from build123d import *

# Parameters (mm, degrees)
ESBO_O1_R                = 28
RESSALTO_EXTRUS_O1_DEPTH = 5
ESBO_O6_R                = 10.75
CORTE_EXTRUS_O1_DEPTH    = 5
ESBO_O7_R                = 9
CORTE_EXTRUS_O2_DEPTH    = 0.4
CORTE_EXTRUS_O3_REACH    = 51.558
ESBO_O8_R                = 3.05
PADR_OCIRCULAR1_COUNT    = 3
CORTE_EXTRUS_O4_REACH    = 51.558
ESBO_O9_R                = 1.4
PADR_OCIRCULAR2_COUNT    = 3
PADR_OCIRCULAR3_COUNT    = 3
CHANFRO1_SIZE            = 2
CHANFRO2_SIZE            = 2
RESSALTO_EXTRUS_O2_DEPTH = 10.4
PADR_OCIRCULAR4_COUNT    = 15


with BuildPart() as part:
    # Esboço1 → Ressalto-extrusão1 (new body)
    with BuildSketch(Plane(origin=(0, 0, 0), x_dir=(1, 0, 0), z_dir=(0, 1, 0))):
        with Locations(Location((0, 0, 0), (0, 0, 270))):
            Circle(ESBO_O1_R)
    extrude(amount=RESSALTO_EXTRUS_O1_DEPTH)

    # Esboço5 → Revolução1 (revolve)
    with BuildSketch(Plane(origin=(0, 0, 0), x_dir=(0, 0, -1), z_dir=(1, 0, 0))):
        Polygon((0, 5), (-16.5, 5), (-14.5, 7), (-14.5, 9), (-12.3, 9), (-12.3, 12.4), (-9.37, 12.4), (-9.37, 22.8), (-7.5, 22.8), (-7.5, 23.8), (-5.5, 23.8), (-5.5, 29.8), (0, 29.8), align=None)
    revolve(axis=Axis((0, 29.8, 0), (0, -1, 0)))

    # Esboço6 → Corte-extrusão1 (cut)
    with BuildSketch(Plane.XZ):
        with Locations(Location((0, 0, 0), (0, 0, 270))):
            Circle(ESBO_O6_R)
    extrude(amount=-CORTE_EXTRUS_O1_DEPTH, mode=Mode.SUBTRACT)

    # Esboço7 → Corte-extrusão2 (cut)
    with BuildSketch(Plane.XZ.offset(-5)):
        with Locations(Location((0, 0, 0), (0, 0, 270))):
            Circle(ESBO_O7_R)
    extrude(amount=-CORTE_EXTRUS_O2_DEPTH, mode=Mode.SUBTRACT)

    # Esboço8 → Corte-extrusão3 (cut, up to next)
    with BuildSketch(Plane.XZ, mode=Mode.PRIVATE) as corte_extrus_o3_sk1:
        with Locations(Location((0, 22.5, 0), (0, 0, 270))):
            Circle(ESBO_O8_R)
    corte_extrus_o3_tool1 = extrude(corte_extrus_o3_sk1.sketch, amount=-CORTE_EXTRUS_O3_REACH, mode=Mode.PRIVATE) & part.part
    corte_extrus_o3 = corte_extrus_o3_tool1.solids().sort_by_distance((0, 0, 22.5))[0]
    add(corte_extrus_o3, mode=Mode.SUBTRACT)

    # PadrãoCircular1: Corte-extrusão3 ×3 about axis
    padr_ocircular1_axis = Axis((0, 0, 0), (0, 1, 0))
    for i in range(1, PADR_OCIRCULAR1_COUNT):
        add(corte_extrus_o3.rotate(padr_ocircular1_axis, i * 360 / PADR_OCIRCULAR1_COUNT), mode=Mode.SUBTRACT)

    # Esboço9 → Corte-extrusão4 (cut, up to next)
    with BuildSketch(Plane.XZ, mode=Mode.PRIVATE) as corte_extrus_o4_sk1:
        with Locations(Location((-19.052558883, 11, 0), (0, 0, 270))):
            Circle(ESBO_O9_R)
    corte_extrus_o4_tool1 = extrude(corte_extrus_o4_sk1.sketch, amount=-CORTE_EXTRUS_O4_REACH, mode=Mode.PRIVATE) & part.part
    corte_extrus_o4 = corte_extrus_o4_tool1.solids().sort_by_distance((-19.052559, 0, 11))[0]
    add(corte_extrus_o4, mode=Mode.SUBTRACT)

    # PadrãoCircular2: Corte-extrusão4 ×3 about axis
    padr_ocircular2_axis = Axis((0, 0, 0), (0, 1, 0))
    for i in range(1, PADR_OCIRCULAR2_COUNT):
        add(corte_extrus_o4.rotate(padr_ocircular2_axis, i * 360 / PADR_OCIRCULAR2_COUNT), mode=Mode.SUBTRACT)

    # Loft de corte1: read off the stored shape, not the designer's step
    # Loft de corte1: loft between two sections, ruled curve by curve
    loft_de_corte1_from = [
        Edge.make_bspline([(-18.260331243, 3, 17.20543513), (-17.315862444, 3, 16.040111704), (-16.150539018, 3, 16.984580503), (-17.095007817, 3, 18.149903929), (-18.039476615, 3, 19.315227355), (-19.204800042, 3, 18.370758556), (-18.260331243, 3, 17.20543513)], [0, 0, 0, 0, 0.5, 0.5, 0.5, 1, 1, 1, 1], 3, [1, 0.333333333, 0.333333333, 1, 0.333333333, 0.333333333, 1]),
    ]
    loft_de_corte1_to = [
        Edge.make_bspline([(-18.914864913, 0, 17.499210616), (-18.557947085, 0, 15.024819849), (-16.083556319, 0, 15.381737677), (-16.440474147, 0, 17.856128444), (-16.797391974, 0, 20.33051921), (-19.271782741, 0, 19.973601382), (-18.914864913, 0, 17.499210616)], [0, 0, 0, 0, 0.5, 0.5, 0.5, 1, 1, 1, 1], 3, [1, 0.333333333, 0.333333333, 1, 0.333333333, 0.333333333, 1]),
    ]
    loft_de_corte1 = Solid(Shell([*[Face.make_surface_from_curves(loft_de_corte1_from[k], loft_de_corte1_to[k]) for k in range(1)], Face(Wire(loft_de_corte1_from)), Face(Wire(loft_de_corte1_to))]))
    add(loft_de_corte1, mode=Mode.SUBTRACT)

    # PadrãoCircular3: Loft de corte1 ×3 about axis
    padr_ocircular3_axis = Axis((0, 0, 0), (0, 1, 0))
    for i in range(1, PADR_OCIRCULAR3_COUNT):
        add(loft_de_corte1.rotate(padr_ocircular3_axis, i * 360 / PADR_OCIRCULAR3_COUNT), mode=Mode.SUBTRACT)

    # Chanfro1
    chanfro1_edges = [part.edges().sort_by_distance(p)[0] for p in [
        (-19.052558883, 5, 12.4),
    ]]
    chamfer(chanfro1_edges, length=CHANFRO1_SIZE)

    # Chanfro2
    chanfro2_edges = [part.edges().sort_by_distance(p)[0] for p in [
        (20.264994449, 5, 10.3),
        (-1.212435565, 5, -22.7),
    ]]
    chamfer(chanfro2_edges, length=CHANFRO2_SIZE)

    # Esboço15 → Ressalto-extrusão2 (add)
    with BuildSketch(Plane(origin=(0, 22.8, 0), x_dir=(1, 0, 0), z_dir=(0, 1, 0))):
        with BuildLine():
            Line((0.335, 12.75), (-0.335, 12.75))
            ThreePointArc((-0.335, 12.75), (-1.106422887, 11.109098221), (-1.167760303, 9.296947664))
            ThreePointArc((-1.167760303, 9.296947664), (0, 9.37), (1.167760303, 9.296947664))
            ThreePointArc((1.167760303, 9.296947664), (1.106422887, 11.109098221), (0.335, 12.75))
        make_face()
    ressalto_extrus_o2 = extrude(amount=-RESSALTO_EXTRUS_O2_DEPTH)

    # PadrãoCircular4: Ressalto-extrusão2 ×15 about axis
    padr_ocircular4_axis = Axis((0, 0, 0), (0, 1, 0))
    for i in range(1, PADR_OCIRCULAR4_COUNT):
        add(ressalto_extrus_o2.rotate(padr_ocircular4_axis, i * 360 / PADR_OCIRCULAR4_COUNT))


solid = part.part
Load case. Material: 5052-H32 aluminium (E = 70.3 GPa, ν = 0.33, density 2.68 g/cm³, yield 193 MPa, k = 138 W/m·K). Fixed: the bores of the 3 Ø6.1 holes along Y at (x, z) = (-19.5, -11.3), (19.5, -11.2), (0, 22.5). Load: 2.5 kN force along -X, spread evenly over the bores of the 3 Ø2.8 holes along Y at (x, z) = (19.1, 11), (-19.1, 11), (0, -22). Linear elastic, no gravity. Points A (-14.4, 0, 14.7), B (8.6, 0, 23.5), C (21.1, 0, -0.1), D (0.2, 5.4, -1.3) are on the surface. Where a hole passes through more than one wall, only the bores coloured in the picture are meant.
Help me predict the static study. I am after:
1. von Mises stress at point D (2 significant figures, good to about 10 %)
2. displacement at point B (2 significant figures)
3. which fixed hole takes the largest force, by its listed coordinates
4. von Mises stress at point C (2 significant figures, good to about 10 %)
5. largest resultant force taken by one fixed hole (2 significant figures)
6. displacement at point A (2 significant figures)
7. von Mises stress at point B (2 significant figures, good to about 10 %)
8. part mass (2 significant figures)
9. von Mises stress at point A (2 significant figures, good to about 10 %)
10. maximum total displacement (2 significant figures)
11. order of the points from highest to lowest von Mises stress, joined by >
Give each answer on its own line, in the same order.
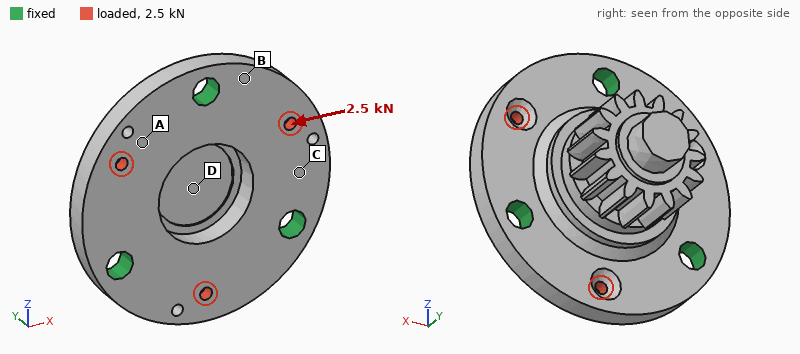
3.8 MPa
1.5 µm
(0, 22.5)
8.6 MPa
1.1 kN
4.7 µm
11 MPa
51 g
18 MPa
9.4 µm
A > B > C > D
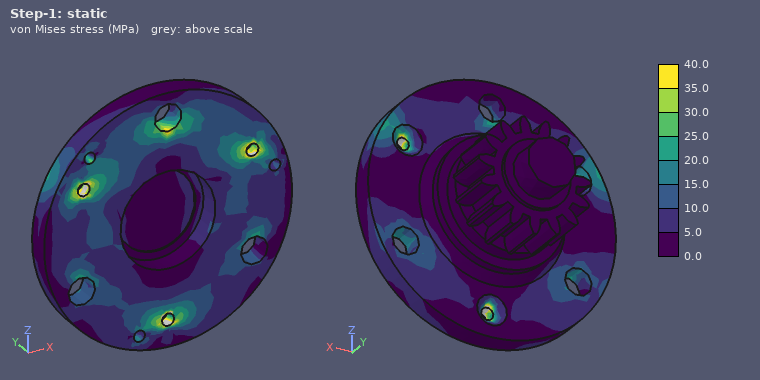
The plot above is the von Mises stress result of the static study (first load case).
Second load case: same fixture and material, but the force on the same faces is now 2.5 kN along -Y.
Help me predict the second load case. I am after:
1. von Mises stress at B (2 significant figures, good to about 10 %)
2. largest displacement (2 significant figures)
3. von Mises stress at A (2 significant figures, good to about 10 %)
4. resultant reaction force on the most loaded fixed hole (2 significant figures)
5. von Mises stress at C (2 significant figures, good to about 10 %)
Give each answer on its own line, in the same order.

25 MPa
37 µm
31 MPa
900 N
29 MPa
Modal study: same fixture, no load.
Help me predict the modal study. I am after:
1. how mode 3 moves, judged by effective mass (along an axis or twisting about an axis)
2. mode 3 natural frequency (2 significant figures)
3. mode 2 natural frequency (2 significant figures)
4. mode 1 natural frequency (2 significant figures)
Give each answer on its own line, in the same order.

along Y
14 kHz
13 kHz
13 kHz
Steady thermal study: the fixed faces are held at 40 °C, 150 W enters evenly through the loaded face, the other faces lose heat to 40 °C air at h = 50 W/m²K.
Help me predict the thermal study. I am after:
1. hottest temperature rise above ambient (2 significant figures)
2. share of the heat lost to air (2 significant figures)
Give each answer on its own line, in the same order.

65 K
6.2 %
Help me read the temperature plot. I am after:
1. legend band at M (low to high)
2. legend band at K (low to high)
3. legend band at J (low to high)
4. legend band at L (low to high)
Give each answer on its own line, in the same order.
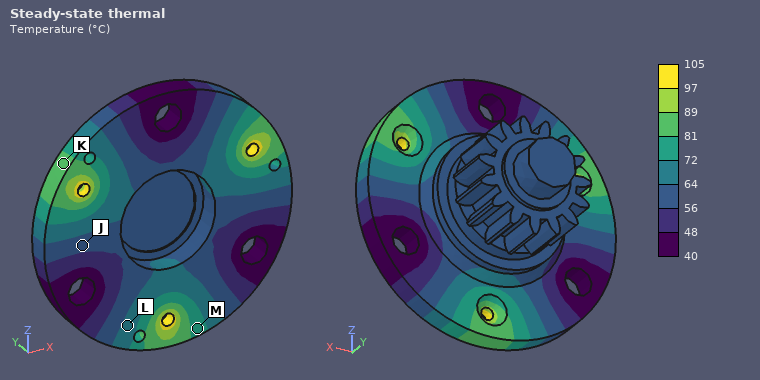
72 to 81 °C
81 to 89 °C
56 to 64 °C
64 to 72 °C
